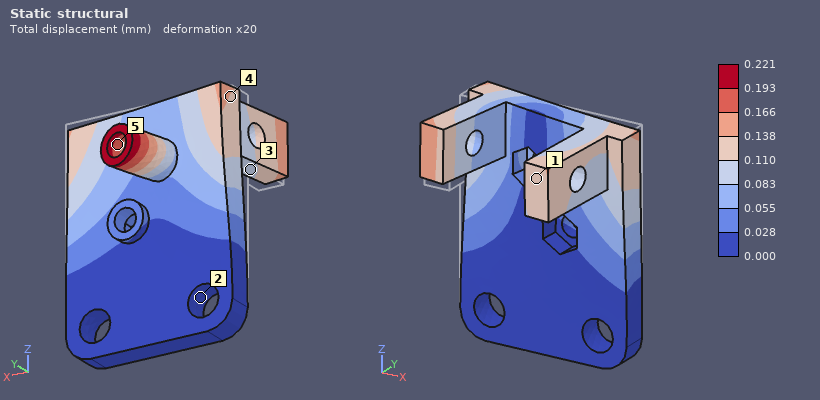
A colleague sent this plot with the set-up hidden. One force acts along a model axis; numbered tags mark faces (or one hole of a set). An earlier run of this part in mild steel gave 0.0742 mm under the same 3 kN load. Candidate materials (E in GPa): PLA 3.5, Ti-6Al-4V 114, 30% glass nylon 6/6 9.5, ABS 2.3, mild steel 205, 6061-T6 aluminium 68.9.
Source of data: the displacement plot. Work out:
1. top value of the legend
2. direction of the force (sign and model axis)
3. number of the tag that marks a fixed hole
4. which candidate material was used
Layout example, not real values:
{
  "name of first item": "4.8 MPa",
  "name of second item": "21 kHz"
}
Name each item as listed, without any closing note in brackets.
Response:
{
  "top value of the legend": "0.221 mm",
  "direction of the force": "+X",
  "number of the tag that marks a fixed hole": "2",
  "which candidate material was used": "6061-T6 aluminium"
}
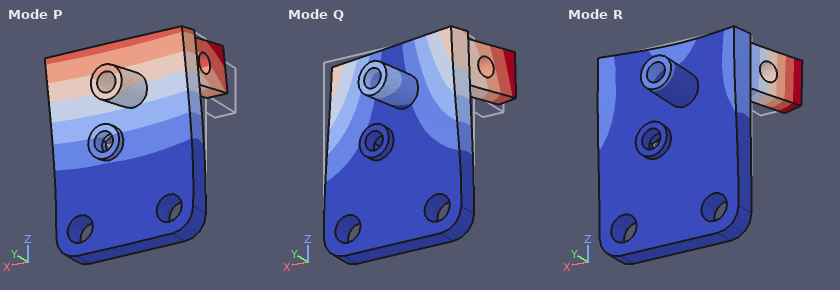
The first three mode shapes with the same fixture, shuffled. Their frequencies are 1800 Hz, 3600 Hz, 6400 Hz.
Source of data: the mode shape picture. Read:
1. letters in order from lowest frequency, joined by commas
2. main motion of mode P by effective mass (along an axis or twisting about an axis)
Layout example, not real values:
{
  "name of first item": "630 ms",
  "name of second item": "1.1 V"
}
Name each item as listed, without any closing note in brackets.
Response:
{
  "letters in order from lowest frequency, joined by commas": "P, Q, R",
  "main motion of mode P by effective mass": "along Y"
}
